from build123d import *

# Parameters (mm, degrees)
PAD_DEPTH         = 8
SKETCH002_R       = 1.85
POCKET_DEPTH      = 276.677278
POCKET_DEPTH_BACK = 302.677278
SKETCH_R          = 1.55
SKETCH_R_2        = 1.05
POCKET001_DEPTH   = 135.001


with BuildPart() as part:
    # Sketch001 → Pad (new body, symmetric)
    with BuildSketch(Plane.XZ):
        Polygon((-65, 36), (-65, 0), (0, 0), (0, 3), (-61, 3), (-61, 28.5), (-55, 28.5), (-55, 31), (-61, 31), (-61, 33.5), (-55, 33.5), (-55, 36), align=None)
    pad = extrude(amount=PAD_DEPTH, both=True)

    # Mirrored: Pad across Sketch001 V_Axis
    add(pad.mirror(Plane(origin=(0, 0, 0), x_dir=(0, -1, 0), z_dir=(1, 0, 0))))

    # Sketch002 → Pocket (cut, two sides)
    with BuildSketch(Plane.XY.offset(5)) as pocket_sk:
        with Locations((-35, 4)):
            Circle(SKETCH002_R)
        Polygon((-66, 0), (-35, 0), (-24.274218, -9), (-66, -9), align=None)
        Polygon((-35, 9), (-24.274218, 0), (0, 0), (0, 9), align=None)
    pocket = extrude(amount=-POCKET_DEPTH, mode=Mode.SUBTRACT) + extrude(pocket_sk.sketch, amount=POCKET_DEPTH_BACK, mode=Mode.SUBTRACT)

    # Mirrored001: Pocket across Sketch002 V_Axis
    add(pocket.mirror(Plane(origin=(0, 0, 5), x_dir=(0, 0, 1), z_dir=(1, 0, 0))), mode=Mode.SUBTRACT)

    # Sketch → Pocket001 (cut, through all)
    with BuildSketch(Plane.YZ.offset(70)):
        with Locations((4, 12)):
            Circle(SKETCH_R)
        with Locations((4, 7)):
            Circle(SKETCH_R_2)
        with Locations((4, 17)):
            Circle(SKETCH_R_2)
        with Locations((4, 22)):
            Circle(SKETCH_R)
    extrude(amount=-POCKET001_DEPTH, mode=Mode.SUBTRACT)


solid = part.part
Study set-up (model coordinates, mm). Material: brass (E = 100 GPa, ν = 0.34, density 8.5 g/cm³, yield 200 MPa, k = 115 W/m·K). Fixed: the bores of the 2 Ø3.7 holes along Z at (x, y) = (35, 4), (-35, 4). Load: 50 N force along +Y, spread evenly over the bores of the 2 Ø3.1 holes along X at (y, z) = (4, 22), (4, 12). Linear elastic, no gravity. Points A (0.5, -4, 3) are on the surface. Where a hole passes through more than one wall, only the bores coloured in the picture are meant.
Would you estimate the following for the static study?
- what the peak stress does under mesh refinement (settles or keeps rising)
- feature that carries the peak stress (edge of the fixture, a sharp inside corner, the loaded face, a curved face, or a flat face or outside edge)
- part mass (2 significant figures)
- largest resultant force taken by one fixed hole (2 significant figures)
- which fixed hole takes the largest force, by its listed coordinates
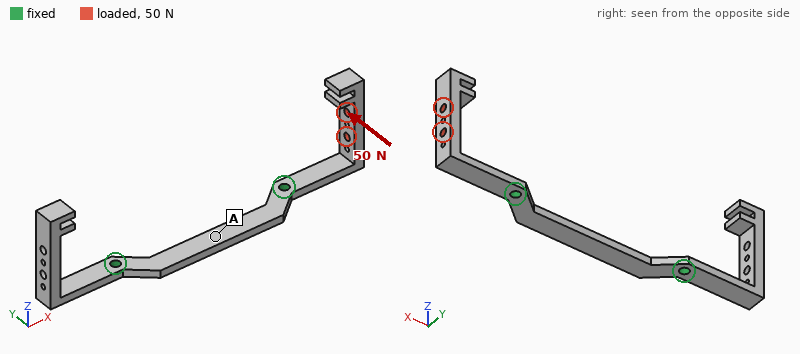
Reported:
keeps rising
edge of the fixture
47 g
53 N
(35, 4)
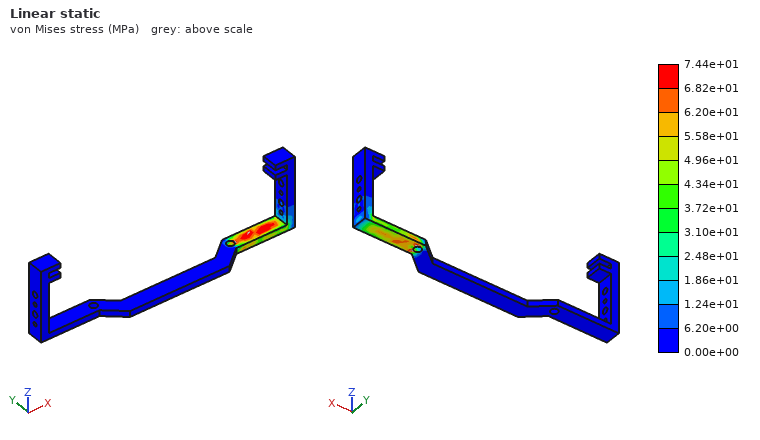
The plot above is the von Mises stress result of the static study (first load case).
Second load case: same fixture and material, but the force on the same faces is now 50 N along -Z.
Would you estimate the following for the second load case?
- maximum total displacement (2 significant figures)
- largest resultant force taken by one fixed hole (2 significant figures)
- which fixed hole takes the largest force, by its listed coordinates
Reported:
0.40 mm
50 N
(35, 4)
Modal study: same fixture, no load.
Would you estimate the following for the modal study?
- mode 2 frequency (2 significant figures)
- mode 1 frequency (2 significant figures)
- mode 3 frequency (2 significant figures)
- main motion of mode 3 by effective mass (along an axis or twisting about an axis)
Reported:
460 Hz
460 Hz
590 Hz
along Y
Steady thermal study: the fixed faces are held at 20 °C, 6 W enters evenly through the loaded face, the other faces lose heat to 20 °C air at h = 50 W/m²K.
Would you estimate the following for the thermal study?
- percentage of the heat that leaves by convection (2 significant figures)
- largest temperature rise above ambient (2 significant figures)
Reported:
48 %
47 K
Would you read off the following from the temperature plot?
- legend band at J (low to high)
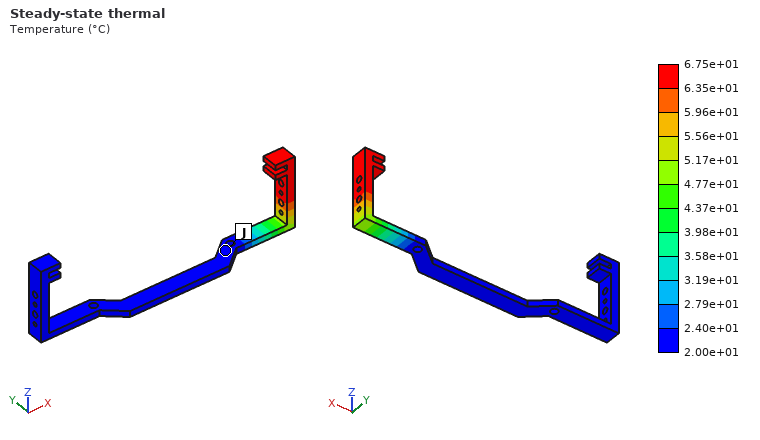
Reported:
2.00e+01 to 2.40e+01 °C
